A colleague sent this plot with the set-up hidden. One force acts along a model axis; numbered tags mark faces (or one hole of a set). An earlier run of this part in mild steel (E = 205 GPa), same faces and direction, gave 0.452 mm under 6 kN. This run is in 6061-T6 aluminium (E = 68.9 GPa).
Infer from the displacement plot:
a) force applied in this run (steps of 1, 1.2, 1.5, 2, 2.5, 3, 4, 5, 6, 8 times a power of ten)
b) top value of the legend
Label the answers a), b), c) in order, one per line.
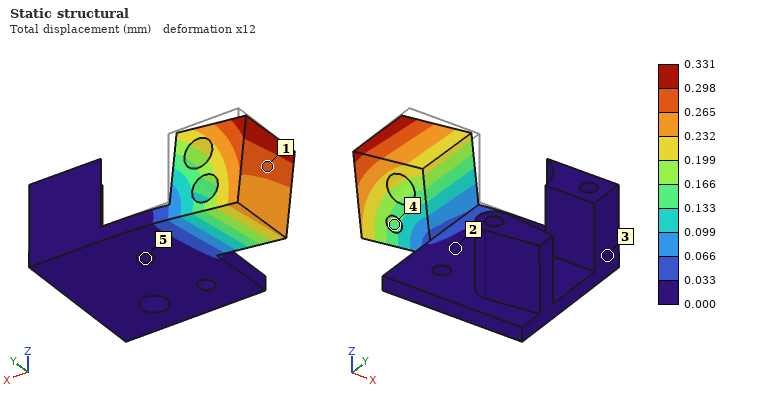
a) 1.5 kN
b) 0.331 mm
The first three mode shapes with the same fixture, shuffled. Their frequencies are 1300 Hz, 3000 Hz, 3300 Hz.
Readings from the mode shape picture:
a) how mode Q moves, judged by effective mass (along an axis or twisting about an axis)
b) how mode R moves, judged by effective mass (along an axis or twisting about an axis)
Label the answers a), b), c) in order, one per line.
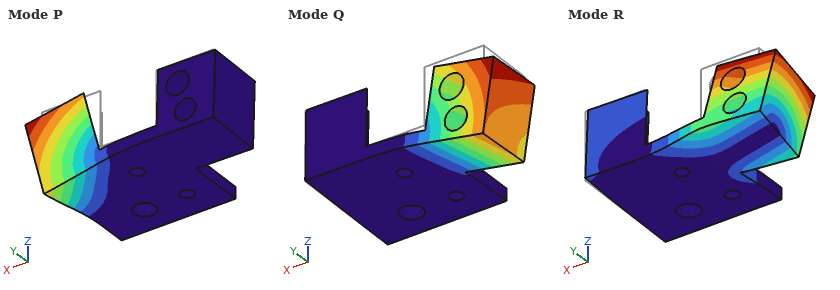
a) along Z
b) along Y
